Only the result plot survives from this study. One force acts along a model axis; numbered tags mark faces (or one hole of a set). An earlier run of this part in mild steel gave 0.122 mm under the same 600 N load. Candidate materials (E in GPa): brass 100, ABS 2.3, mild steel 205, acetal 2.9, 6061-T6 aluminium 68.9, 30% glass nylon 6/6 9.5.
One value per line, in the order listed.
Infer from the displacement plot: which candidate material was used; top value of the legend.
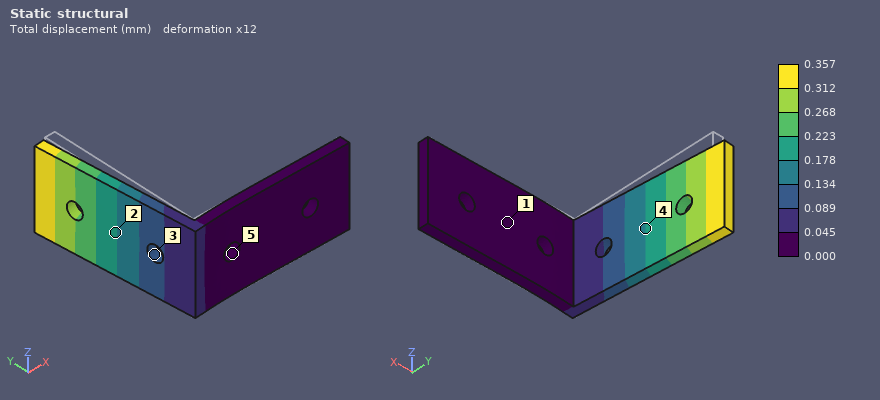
6061-T6 aluminium
0.357 mm
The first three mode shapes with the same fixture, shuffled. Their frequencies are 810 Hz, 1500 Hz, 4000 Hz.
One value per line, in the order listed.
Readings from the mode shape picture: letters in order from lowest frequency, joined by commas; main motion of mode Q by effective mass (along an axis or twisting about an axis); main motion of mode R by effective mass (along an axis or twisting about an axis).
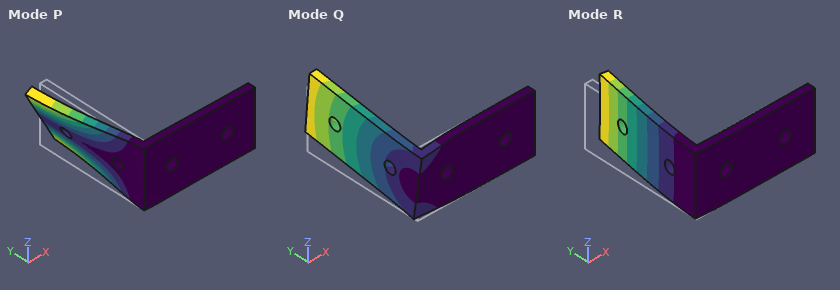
R, Q, P
along Z
along X
